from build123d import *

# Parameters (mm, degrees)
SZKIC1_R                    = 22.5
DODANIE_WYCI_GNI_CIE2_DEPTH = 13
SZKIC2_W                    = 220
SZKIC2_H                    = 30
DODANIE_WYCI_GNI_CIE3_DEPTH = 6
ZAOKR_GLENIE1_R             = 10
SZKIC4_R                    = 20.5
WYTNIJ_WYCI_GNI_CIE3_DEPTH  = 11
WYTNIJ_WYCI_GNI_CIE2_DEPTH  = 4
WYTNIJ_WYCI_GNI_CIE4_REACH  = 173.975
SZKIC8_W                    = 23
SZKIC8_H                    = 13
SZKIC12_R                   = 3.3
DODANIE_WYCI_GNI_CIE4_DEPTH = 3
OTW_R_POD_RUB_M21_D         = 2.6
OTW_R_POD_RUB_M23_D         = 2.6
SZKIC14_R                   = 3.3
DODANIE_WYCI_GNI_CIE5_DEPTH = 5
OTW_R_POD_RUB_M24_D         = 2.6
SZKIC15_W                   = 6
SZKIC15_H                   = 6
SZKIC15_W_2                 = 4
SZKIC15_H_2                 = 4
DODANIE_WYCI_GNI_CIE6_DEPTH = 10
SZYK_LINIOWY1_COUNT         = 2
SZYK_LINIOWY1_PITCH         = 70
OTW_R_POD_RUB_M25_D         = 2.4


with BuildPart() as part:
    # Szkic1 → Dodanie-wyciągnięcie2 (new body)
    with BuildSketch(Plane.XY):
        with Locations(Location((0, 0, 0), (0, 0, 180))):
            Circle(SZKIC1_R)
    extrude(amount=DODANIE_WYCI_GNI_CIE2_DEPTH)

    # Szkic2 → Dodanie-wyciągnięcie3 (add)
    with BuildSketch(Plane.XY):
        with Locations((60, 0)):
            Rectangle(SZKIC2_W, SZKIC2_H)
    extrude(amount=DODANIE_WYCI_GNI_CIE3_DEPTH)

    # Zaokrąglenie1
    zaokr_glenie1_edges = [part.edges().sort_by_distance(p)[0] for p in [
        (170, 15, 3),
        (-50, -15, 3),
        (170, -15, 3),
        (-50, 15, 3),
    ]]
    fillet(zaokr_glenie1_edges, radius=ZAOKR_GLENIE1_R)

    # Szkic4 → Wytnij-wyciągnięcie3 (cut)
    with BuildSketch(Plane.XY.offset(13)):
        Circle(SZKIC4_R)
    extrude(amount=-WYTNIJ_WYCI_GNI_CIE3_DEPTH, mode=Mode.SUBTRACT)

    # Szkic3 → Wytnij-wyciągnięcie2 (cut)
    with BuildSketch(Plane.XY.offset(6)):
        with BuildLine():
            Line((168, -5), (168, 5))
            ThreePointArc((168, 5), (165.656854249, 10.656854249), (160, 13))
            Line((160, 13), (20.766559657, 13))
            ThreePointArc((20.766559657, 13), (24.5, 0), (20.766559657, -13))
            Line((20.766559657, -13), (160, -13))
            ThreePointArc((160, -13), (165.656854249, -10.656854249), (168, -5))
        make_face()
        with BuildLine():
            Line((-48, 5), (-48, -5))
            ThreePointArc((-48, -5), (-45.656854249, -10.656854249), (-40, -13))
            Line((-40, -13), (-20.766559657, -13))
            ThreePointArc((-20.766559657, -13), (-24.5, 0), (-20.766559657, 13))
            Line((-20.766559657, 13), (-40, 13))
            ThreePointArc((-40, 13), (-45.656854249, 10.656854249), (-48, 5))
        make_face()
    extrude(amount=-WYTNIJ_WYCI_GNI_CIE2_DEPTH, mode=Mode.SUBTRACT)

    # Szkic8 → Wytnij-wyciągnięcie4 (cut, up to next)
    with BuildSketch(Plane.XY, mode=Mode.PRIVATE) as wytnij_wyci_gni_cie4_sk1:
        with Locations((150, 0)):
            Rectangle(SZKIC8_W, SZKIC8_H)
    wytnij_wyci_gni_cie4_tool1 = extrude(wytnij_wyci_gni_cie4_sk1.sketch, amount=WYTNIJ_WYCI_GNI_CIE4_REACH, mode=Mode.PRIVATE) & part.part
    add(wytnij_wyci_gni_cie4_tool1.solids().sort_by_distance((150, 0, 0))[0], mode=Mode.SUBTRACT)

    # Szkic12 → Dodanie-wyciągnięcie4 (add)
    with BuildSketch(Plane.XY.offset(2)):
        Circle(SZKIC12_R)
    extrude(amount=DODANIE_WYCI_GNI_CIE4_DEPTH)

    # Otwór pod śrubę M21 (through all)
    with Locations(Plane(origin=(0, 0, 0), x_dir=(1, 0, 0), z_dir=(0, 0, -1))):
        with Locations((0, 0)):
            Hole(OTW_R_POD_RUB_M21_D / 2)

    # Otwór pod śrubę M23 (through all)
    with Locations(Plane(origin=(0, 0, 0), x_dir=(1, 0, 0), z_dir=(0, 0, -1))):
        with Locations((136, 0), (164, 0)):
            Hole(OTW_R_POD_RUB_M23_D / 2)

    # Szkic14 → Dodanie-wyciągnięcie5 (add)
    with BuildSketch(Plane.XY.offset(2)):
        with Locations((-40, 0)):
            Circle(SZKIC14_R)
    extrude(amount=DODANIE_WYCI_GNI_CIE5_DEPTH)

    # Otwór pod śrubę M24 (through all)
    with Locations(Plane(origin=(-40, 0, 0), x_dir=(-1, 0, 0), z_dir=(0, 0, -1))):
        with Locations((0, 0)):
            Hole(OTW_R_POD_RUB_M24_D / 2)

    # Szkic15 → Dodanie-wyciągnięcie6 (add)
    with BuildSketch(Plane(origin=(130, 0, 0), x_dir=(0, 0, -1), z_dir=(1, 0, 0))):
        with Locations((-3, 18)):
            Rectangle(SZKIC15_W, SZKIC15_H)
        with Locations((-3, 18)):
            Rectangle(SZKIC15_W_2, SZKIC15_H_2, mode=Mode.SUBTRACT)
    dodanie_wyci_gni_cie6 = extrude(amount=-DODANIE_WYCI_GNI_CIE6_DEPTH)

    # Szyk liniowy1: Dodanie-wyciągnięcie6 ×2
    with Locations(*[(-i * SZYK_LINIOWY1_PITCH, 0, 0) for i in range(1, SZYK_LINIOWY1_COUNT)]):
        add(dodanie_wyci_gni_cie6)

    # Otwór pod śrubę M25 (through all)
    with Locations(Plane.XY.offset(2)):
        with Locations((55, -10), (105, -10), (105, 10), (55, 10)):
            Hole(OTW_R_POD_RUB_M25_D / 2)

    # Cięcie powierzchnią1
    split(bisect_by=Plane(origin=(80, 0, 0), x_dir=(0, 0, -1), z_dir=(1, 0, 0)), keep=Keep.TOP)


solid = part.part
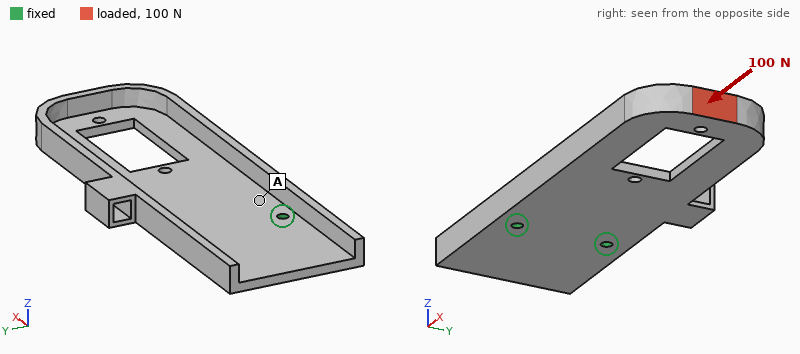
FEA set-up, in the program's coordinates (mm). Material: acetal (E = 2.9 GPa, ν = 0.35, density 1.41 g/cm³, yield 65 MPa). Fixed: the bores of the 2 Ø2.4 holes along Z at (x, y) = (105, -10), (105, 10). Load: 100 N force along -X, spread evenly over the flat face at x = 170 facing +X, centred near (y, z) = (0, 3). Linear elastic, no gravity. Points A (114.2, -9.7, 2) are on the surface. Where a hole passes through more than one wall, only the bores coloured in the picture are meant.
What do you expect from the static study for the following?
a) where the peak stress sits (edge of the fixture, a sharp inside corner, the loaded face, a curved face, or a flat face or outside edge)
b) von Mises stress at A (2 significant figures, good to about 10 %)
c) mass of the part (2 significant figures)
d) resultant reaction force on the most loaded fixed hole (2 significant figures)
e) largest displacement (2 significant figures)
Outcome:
a curved face
1.9 MPa
9.1 g
50 N
1.2 mm
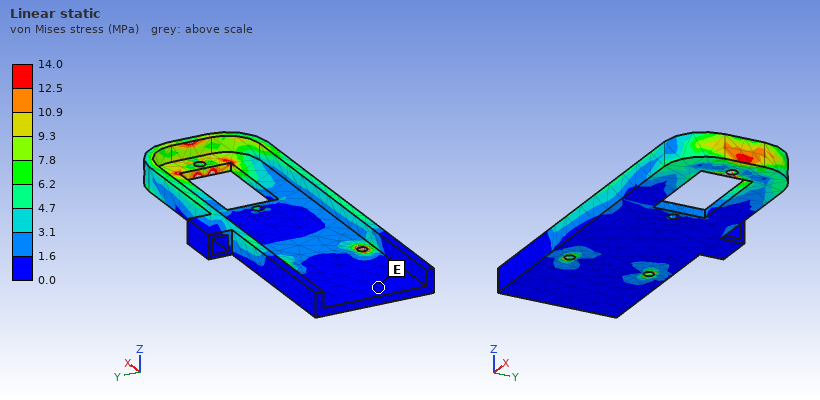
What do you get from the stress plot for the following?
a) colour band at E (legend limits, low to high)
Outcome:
0.0 to 1.6 MPa
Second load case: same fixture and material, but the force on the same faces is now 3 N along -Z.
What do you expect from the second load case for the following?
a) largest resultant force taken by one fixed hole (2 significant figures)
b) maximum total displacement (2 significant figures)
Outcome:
2.1 N
1.0 mm
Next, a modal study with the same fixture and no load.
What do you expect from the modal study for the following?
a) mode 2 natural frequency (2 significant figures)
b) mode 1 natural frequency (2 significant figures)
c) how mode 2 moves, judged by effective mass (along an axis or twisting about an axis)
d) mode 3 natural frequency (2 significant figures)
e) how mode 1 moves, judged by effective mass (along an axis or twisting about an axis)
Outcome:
520 Hz
210 Hz
twisting about X
1100 Hz
along Z
